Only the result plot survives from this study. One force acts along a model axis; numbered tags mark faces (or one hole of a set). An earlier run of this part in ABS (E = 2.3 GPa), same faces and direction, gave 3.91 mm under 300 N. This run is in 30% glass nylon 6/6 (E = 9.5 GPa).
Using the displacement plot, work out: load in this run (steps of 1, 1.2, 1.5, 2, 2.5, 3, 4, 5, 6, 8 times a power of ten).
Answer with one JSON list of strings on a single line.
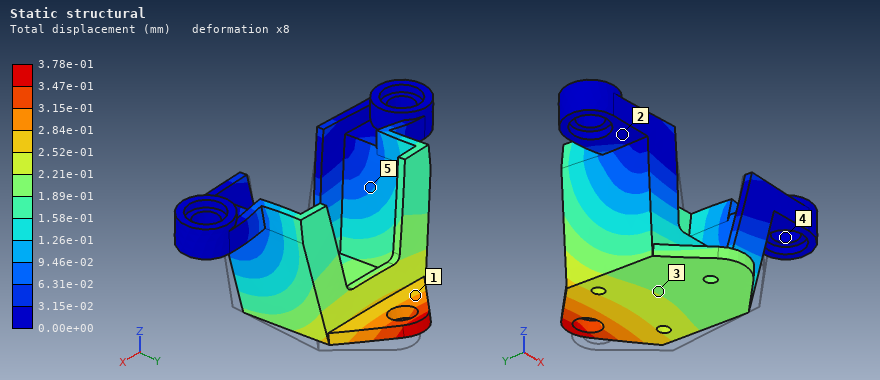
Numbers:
["120 N"]
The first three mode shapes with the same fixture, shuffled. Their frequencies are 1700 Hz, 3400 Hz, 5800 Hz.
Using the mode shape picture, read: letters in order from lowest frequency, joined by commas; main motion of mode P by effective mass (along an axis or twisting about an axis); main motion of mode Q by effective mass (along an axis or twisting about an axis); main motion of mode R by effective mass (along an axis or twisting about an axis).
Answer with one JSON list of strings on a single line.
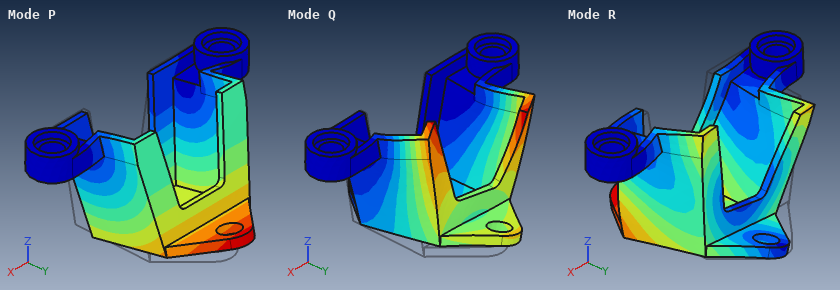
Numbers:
["P, Q, R", "along Y", "along X", "along X"]
